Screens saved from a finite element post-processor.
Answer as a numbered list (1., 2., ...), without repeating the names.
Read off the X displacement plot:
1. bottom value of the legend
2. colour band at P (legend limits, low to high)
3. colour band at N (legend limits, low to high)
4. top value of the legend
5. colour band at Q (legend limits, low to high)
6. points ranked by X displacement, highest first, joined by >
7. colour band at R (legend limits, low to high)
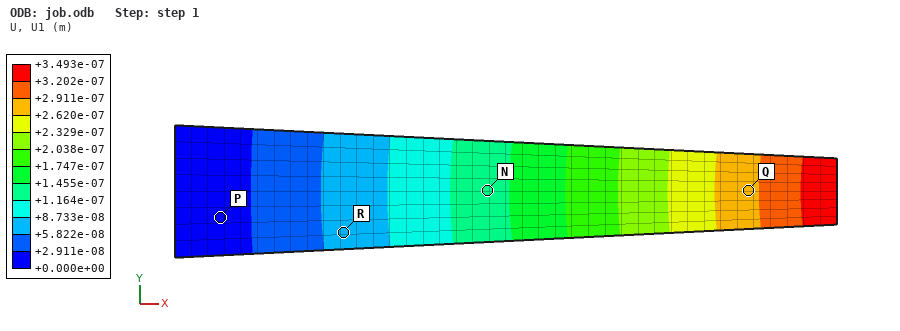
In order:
1. +0.000e+00 m
2. +0.000e+00 to +2.911e-08 m
3. +1.164e-07 to +1.455e-07 m
4. +3.493e-07 m
5. +2.620e-07 to +2.911e-07 m
6. Q > N > R > P
7. +5.822e-08 to +8.733e-08 m
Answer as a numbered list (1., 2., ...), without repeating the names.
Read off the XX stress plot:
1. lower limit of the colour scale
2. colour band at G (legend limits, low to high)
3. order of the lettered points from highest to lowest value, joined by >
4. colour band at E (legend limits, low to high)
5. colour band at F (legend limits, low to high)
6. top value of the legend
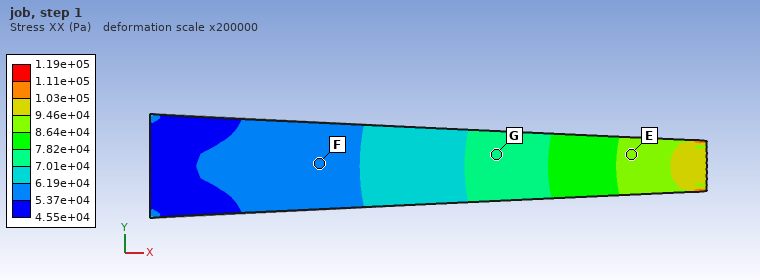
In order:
1. 4.55e+04 Pa
2. 7.01e+04 to 7.82e+04 Pa
3. E > G > F
4. 8.64e+04 to 9.46e+04 Pa
5. 5.37e+04 to 6.19e+04 Pa
6. 1.19e+05 Pa
